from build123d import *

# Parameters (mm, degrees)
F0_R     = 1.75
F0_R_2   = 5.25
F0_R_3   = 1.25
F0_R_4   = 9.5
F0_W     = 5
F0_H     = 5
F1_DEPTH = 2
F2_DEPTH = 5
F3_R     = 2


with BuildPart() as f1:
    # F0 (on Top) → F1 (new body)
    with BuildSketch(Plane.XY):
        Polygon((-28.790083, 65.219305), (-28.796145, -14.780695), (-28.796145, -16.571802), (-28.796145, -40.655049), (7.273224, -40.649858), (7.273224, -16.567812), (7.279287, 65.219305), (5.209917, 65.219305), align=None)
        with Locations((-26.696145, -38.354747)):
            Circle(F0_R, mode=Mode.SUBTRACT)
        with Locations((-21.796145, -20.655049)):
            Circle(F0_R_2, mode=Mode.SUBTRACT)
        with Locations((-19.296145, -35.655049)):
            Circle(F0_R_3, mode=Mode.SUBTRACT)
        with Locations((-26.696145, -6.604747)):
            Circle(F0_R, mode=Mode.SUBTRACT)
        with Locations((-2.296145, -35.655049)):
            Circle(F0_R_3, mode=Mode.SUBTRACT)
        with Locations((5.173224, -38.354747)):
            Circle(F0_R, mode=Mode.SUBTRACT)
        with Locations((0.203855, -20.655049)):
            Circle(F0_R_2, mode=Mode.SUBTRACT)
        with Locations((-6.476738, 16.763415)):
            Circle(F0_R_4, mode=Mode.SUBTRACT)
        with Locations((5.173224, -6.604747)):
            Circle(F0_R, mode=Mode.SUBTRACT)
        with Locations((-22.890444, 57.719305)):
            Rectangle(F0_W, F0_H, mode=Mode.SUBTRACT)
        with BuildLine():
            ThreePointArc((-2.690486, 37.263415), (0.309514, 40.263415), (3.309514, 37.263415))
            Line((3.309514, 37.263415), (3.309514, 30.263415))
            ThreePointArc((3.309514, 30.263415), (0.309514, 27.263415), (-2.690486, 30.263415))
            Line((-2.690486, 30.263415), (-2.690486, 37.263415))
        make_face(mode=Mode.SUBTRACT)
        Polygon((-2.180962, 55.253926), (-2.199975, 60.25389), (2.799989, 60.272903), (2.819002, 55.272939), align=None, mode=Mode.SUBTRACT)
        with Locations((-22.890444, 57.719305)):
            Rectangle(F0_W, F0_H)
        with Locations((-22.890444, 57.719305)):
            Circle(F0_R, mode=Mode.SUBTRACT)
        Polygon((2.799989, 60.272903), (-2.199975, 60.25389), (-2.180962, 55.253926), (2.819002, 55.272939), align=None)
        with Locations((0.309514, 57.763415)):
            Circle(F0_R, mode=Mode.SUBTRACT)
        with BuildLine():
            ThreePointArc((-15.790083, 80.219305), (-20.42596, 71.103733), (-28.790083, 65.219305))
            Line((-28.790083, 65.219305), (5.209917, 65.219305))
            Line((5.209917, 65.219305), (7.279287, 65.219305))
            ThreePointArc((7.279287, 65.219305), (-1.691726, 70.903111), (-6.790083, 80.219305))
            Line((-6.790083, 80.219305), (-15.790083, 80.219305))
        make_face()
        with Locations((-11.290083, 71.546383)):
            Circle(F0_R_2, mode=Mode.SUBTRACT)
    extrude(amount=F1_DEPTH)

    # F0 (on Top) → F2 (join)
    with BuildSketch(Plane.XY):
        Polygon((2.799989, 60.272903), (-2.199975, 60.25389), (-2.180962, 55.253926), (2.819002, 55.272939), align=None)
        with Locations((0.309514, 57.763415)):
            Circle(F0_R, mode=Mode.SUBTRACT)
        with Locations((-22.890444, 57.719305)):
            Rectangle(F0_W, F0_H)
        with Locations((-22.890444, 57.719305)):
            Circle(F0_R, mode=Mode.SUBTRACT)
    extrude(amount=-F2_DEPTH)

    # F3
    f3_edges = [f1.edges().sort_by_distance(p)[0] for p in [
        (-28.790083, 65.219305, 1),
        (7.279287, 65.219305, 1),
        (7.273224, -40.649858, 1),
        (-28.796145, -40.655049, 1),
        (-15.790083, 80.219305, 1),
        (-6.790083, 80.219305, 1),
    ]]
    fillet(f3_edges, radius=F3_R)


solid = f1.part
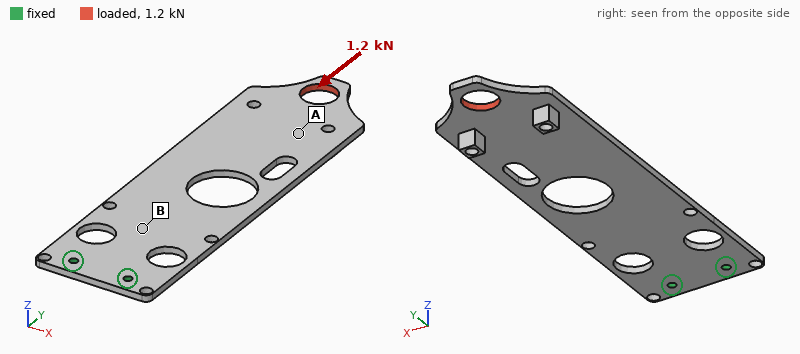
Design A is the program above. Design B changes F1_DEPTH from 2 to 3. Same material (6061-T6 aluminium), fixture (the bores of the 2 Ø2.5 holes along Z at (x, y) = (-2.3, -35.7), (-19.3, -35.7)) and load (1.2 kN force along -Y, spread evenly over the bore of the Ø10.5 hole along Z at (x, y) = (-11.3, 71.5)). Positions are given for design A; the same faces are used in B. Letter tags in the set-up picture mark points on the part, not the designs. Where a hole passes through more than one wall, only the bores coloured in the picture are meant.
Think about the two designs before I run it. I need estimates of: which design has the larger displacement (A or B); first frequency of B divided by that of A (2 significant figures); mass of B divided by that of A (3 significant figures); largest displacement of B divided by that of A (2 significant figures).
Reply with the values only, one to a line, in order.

A
1.5
1.49
0.66
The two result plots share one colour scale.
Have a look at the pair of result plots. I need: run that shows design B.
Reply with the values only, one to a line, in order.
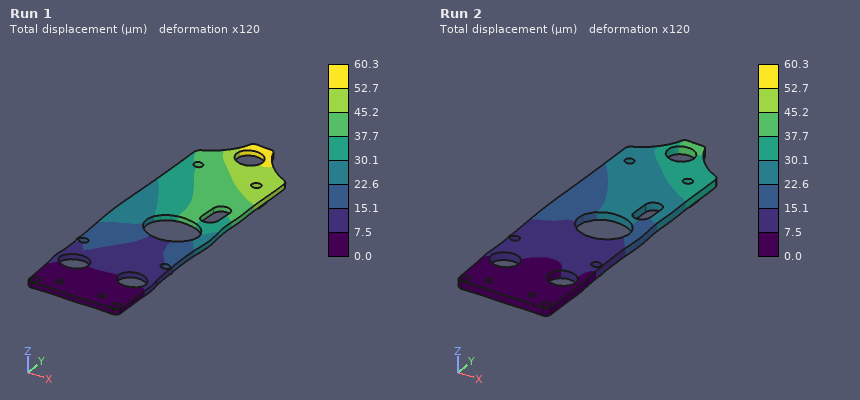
Run 2
